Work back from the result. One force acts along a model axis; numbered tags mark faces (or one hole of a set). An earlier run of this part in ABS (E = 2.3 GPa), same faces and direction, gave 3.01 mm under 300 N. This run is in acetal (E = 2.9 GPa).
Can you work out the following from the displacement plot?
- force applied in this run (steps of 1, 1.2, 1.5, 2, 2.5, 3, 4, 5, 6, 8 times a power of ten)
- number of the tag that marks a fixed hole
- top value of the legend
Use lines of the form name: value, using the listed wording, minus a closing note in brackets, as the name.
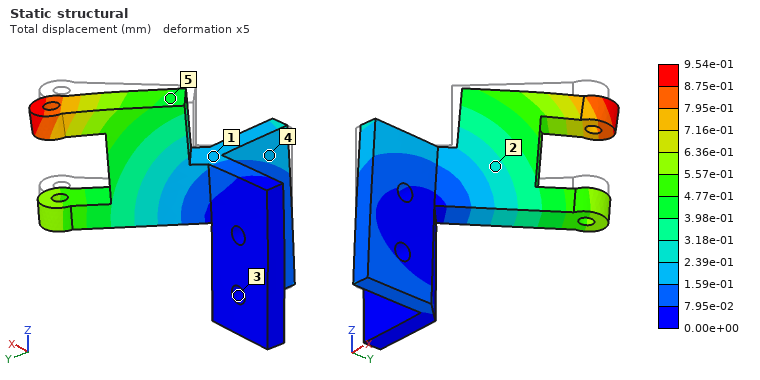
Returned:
force applied in this run: 120 N
number of the tag that marks a fixed hole: 3
top value of the legend: 9.54e-01 mm
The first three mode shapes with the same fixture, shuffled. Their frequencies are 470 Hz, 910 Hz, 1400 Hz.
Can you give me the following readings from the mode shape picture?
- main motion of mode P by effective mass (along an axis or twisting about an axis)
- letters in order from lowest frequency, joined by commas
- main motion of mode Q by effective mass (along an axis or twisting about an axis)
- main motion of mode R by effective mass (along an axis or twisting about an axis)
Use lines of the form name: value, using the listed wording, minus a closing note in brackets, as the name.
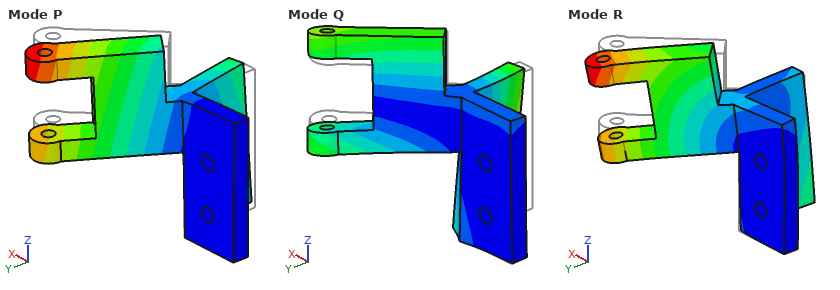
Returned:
main motion of mode P by effective mass: along Y
letters in order from lowest frequency, joined by commas: P, R, Q
main motion of mode Q by effective mass: along X
main motion of mode R by effective mass: along Z
